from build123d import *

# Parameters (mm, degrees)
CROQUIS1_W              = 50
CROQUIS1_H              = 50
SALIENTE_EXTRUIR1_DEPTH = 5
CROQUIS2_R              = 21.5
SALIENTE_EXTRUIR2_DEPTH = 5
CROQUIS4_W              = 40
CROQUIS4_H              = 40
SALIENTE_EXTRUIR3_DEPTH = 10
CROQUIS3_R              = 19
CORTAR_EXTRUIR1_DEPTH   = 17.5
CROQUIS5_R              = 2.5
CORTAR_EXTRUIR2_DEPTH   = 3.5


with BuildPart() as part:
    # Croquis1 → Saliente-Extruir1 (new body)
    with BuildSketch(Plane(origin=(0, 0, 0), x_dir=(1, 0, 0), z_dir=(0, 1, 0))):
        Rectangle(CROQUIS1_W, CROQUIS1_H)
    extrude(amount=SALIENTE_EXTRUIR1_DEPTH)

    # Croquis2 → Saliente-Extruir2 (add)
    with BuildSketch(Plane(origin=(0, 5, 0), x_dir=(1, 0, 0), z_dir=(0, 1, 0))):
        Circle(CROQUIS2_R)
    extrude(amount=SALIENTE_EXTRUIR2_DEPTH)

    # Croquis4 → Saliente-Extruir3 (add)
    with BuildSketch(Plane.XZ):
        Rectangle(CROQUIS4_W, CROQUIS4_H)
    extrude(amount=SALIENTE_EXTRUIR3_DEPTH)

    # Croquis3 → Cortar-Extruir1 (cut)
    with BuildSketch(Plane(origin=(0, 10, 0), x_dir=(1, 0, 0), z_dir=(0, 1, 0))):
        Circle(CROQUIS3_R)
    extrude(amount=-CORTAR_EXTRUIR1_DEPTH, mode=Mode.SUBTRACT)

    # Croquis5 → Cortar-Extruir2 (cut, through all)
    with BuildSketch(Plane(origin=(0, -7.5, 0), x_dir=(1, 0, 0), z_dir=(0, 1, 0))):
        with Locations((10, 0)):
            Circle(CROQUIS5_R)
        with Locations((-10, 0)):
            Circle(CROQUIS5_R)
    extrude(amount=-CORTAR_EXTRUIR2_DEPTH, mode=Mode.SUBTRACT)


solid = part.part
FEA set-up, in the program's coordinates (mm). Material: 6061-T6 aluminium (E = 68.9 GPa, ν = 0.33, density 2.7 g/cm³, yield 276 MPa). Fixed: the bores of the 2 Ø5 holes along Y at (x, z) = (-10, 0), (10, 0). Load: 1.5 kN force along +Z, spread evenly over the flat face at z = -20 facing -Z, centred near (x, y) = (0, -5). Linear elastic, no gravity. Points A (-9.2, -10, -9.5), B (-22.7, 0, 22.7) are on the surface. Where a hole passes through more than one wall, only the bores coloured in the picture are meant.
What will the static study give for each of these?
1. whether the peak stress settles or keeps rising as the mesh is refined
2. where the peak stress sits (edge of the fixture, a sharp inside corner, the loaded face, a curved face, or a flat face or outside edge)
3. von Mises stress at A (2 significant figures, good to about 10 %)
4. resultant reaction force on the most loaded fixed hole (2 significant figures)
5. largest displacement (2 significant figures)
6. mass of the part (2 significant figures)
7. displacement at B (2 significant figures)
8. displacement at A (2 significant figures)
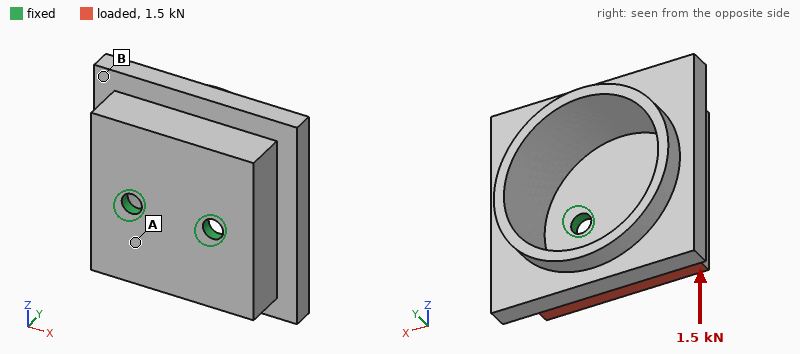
keeps rising
edge of the fixture
20 MPa
760 N
92 µm
43 g
73 µm
20 µm
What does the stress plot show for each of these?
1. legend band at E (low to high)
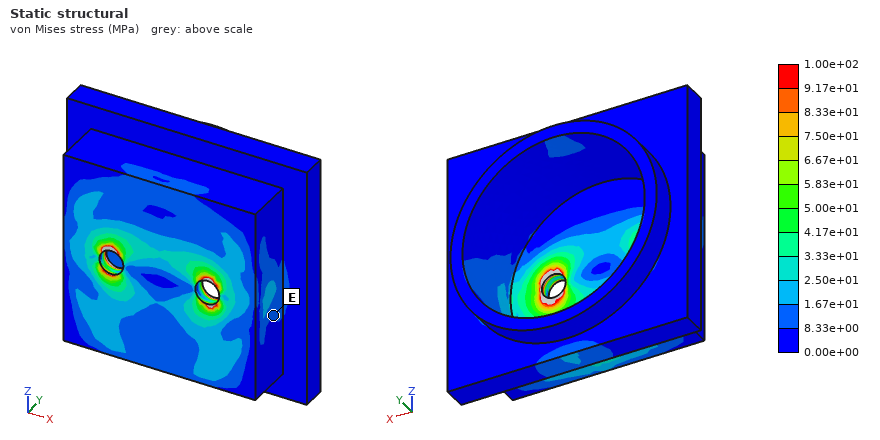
8.33e+00 to 1.67e+01 MPa
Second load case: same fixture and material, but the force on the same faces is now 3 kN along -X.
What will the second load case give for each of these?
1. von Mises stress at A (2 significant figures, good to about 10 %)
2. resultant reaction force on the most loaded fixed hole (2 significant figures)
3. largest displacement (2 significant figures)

51 MPa
2.9 kN
87 µm
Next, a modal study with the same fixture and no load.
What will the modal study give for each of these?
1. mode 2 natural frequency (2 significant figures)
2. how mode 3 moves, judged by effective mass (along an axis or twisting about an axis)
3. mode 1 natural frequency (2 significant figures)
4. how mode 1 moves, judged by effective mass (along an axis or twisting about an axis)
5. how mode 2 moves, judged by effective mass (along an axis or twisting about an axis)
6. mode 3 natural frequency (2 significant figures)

4100 Hz
along Y
1900 Hz
along Z
along X
5500 Hz
